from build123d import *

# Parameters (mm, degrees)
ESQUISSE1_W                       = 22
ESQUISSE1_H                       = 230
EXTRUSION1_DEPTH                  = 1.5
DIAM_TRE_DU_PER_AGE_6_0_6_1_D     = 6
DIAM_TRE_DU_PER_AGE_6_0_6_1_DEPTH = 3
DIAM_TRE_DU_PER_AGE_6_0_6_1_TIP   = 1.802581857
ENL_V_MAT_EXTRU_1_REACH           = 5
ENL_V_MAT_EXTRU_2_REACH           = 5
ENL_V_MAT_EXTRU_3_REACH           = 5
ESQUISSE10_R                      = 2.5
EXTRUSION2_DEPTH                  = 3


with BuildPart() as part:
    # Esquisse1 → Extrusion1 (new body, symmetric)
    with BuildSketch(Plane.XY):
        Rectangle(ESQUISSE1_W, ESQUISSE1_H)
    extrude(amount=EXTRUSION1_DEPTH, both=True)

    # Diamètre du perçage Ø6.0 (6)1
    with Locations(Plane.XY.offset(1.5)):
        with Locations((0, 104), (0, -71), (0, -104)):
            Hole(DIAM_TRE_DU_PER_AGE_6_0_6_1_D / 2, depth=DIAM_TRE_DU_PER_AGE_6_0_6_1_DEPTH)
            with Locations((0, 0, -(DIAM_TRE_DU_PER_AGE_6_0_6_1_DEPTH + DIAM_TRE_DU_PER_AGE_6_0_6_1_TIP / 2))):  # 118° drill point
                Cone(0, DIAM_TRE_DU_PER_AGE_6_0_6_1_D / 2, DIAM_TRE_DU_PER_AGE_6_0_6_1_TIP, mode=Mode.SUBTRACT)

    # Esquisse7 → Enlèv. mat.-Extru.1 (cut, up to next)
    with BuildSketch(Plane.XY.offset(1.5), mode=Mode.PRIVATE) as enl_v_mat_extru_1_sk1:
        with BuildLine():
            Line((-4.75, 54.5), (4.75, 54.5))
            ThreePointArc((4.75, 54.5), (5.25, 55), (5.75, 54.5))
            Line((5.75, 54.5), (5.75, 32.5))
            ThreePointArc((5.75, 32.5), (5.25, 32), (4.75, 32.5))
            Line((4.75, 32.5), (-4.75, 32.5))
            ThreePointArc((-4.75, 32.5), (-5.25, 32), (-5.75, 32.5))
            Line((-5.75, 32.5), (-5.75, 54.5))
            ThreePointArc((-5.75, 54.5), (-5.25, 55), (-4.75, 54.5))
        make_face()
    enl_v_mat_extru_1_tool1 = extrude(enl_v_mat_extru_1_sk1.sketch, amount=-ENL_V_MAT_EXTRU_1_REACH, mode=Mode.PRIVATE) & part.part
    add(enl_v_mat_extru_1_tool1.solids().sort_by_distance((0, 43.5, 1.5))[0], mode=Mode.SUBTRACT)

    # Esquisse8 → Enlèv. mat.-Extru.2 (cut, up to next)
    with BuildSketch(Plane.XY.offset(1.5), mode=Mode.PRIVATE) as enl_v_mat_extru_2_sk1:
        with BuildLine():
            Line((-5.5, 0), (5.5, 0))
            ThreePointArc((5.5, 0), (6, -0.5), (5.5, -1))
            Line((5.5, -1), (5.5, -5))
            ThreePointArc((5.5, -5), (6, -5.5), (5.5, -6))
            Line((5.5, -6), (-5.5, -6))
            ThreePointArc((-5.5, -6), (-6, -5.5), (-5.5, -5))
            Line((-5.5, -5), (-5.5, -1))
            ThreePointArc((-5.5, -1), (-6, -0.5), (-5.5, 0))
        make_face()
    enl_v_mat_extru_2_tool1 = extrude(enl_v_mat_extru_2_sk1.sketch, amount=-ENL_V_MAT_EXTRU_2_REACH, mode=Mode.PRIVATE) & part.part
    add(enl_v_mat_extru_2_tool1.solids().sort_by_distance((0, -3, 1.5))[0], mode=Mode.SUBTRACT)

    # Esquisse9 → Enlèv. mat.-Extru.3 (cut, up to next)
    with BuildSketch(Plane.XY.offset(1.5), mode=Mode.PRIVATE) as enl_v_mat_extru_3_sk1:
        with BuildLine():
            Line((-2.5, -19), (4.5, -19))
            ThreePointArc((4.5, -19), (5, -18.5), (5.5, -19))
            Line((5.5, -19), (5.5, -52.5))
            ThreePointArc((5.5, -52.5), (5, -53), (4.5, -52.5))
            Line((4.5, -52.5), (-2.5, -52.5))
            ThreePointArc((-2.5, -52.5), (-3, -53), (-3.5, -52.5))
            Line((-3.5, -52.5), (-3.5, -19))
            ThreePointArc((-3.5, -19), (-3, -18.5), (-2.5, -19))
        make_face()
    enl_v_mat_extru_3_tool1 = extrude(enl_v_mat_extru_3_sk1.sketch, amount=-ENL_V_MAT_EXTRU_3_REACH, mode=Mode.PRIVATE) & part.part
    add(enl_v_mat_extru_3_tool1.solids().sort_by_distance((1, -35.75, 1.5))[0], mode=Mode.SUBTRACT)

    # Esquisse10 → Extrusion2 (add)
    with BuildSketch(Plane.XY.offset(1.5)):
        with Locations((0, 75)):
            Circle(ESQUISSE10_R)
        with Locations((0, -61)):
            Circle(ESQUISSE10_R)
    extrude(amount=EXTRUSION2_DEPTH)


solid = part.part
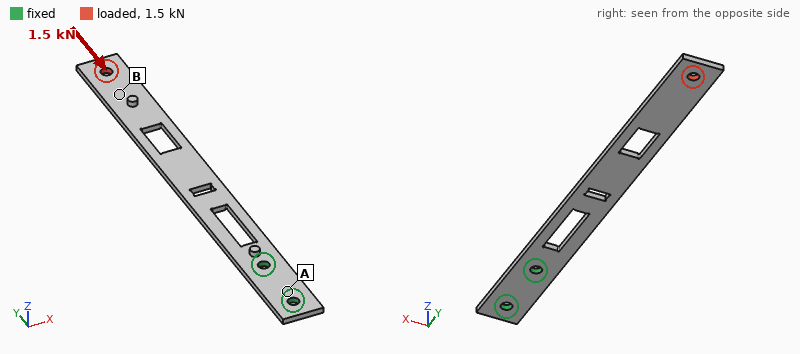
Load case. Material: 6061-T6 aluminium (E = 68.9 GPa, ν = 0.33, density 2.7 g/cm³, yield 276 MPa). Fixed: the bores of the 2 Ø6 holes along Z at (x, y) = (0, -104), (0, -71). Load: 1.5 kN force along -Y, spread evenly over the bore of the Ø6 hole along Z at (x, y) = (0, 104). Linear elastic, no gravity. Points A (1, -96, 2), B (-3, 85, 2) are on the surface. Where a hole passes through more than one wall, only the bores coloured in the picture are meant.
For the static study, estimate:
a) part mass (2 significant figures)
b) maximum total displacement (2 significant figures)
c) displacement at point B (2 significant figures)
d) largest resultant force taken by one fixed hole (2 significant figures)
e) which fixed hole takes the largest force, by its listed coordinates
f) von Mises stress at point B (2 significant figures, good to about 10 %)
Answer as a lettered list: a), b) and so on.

a) 36 g
b) 99 µm
c) 86 µm
d) 1.4 kN
e) (0, -71)
f) 23 MPa
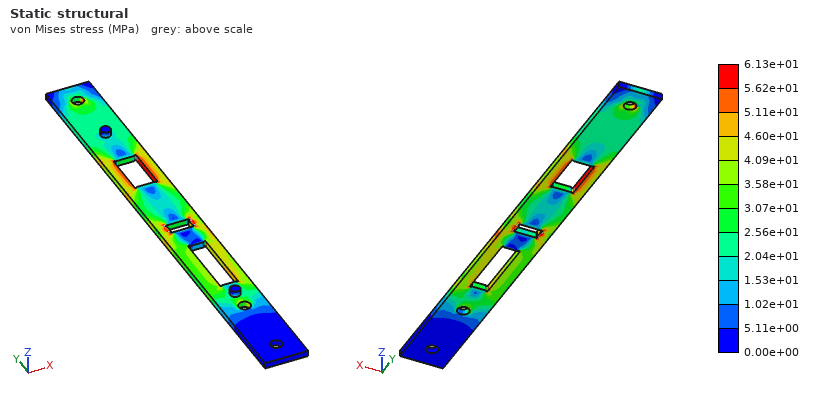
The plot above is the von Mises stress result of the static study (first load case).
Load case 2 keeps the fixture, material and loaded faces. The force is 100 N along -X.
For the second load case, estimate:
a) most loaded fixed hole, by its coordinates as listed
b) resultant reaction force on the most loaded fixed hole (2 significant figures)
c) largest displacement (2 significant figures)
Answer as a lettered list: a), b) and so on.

a) (0, -71)
b) 410 N
c) 1.4 mm
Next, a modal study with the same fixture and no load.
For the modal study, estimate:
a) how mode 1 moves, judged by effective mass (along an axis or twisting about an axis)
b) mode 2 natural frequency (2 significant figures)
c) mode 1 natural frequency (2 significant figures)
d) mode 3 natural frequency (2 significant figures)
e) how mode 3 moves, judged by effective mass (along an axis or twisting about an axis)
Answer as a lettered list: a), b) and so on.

a) along Z
b) 410 Hz
c) 63 Hz
d) 450 Hz
e) along X
